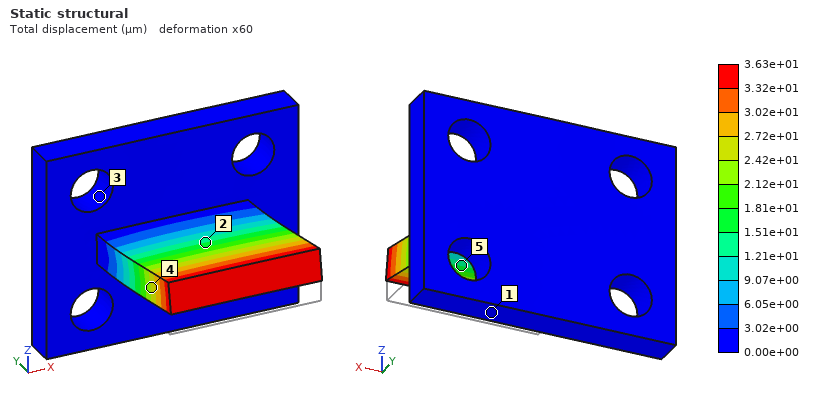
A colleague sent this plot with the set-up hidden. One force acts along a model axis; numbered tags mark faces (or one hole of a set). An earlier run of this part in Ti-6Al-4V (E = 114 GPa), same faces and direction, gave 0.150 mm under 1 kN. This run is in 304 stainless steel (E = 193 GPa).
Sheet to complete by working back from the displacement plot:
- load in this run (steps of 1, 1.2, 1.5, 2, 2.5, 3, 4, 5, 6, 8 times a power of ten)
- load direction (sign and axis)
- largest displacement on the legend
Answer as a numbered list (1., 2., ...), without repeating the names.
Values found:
1. 400 N
2. +Z
3. 3.63e+01 µm
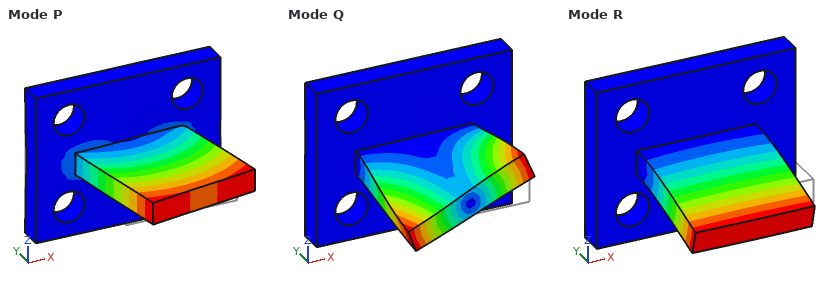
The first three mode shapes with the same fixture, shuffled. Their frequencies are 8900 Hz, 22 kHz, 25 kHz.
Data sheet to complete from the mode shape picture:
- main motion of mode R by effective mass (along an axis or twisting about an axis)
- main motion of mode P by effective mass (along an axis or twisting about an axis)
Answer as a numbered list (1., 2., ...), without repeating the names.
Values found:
1. along Z
2. along X
